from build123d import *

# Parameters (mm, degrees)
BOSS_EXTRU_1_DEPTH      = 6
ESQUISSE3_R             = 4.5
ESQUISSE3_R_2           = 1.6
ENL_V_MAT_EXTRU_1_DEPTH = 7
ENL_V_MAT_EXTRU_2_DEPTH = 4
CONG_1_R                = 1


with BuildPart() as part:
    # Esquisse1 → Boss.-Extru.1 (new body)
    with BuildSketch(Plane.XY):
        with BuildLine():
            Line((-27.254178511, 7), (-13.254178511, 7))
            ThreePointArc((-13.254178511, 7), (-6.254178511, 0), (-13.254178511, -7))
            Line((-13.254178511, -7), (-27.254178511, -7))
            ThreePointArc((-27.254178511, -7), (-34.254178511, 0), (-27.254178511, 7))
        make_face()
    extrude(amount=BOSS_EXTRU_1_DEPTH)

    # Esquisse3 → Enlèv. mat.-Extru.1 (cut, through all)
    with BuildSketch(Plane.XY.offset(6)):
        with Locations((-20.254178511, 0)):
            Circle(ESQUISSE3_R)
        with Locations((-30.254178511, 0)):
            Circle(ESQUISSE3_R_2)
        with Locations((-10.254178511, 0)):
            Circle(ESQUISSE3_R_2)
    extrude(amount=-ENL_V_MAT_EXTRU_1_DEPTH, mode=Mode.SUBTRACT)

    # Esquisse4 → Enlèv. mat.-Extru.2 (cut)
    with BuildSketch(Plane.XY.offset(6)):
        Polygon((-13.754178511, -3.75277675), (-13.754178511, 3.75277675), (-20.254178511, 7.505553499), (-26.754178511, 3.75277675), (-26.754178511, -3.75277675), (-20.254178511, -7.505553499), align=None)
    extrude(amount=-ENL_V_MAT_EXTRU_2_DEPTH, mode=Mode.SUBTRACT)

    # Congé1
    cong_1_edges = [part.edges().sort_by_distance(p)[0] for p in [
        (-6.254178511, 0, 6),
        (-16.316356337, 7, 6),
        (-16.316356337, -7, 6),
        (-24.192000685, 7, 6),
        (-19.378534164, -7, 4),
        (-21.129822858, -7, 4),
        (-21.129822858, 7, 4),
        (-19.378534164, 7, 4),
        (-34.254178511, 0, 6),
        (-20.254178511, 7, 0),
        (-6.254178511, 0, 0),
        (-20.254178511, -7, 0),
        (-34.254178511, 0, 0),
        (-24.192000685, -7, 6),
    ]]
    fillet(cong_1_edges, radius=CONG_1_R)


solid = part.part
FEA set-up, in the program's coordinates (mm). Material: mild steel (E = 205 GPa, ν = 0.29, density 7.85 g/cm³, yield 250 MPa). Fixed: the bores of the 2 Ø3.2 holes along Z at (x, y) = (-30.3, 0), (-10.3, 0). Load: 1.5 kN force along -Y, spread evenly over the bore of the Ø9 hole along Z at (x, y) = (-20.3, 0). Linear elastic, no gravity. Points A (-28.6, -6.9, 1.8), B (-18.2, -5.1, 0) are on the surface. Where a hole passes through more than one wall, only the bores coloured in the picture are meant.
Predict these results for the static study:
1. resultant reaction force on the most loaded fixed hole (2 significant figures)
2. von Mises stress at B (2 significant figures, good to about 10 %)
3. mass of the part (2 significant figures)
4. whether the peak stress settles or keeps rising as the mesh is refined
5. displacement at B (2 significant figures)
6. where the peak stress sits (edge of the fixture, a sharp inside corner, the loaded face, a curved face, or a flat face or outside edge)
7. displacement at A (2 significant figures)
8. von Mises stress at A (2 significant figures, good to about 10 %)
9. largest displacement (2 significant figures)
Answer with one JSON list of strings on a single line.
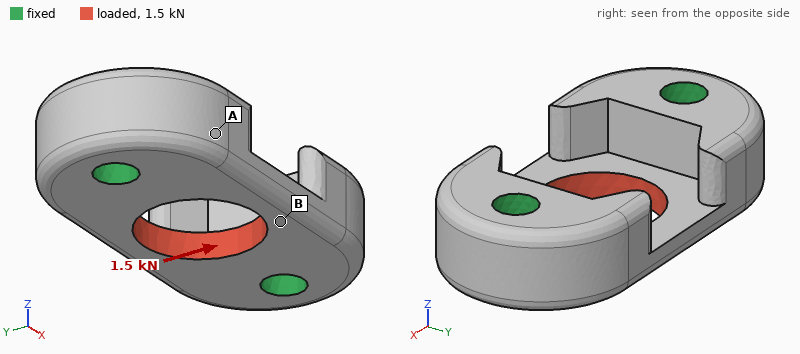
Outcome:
["750 N", "57 MPa", "9.6 g", "keeps rising", "4.1 µm", "edge of the fixture", "1.4 µm", "16 MPa", "4.9 µm"]
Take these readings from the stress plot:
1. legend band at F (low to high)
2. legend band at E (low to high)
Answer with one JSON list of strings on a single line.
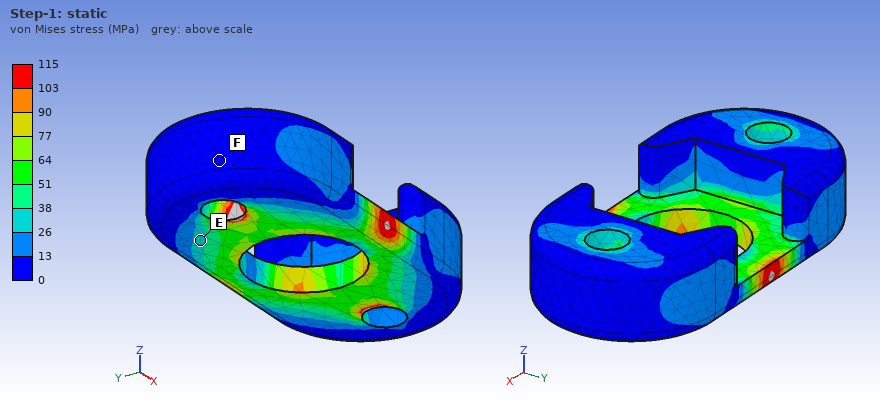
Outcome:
["0 to 13 MPa", "26 to 38 MPa"]
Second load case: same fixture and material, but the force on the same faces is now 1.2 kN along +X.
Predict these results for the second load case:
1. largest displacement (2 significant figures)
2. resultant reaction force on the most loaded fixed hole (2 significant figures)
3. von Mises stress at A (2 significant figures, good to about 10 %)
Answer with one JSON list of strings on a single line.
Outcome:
["1.5 µm", "600 N", "6.2 MPa"]
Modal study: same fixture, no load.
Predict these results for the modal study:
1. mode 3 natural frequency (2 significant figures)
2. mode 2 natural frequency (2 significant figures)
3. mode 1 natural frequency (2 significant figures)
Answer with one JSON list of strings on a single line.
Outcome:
["65 kHz", "56 kHz", "54 kHz"]
